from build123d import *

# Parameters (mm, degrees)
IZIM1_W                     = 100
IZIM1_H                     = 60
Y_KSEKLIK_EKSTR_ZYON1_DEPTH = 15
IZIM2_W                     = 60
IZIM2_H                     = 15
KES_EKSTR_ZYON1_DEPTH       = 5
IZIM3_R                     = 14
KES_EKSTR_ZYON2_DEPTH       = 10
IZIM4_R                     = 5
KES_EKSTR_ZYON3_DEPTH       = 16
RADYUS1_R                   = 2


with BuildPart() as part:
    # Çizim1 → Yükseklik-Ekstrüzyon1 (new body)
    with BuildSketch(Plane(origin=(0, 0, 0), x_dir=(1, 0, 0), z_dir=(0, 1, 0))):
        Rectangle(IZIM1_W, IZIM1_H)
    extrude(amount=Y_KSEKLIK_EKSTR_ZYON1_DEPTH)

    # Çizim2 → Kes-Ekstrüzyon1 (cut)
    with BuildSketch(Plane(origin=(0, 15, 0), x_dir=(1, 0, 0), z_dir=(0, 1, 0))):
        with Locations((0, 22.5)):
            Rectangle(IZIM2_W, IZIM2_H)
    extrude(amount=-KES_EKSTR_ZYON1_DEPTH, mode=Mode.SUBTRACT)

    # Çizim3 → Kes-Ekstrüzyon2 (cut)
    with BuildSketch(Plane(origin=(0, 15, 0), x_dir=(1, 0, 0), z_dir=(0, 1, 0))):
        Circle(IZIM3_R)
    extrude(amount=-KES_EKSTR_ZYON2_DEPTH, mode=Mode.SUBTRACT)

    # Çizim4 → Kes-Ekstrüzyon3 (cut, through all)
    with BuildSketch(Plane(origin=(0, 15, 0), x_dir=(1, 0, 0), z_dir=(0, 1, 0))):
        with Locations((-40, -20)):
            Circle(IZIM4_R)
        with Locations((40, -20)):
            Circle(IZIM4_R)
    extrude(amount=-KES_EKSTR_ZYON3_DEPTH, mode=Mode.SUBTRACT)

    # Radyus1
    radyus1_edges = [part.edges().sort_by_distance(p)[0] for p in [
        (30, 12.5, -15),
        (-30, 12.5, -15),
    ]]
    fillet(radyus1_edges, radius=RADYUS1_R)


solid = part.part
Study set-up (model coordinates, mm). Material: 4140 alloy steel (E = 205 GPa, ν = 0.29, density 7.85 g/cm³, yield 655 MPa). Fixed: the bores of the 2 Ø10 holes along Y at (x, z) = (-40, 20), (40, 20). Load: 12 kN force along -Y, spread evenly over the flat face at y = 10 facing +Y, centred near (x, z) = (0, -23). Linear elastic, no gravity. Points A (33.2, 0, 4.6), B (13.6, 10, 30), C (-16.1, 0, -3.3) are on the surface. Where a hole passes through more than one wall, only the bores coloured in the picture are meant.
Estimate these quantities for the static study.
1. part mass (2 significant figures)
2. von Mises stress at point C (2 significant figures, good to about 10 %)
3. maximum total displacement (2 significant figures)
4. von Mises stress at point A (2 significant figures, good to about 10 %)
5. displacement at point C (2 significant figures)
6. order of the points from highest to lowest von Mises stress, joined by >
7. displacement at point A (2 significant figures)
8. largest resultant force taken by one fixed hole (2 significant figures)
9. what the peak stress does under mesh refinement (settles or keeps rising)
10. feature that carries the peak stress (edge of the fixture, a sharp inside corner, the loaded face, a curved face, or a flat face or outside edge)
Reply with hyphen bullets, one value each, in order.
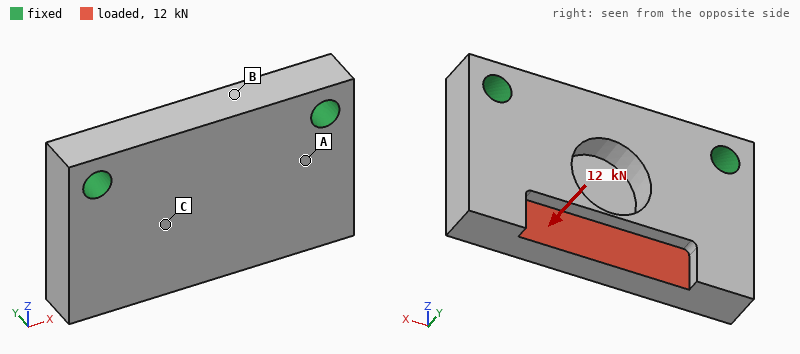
- 600 g
- 75 MPa
- 0.16 mm
- 130 MPa
- 0.057 mm
- A > C > B
- 0.025 mm
- 6.1 kN
- keeps rising
- edge of the fixture
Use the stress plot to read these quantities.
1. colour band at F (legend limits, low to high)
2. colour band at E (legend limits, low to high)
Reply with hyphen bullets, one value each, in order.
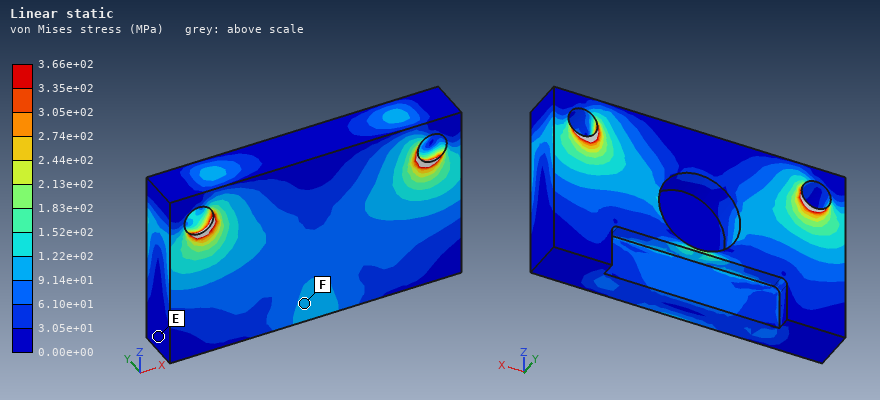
- 9.14e+01 to 1.22e+02 MPa
- 0.00e+00 to 3.05e+01 MPa
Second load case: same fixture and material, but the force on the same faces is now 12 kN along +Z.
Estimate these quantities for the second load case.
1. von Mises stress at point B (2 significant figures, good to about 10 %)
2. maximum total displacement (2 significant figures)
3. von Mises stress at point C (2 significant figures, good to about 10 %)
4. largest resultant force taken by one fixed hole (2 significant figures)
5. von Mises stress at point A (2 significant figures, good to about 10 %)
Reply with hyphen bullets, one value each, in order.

- 7.4 MPa
- 21 µm
- 13 MPa
- 6.5 kN
- 14 MPa
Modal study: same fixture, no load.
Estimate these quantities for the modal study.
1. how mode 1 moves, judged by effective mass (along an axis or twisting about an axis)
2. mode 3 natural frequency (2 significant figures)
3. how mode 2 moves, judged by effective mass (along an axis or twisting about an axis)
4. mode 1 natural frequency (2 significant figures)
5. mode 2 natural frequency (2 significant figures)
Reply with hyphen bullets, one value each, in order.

- along Y
- 9300 Hz
- twisting about Z
- 4100 Hz
- 6400 Hz
